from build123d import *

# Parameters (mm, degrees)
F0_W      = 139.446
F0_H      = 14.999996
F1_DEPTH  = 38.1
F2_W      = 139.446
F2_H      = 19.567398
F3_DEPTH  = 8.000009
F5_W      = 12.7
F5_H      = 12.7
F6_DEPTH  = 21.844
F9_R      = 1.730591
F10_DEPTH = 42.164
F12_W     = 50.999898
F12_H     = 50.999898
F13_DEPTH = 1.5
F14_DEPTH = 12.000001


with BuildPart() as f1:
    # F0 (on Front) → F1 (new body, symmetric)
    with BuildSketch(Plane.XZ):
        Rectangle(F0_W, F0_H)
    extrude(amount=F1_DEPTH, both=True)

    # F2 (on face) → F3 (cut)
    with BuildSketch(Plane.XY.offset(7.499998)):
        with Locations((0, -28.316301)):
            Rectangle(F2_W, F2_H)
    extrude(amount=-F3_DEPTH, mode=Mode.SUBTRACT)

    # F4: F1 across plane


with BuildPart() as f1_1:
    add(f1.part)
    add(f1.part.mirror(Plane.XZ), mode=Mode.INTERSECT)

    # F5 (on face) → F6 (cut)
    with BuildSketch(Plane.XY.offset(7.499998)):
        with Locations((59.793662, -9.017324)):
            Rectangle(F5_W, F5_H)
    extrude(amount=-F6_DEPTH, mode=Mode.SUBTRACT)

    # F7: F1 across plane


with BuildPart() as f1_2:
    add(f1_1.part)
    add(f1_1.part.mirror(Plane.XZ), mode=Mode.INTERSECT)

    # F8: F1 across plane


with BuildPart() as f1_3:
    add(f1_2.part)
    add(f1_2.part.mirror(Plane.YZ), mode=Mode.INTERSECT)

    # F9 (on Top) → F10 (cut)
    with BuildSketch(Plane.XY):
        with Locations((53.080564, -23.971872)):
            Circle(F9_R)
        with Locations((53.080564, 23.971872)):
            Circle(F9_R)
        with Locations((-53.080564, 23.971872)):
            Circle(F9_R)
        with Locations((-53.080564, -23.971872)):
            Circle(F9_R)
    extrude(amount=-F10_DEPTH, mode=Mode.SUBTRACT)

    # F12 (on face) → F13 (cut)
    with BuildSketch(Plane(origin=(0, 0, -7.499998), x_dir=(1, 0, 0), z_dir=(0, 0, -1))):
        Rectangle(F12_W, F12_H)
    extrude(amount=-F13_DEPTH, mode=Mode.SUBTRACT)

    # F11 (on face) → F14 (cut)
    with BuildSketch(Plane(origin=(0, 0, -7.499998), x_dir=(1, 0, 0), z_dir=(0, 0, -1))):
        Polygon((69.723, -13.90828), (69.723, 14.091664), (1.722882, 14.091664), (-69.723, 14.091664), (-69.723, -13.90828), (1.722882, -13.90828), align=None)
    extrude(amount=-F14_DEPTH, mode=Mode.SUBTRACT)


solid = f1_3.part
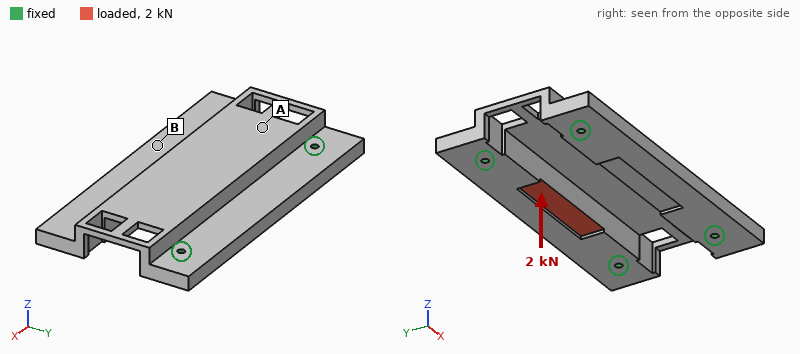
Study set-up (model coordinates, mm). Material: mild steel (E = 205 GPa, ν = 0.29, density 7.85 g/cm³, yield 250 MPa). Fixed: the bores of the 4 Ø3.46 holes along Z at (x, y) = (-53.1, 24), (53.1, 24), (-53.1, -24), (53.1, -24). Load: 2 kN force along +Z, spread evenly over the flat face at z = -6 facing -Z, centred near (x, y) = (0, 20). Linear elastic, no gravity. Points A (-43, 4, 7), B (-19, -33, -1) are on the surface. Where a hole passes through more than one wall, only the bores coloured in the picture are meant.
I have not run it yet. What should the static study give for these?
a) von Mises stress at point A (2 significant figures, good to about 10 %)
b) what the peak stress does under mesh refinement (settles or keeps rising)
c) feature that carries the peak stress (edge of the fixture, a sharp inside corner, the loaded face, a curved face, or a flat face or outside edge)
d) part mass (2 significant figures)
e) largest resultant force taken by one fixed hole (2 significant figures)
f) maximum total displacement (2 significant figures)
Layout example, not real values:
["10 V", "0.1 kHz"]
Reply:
["15 MPa", "keeps rising", "edge of the fixture", "500 g", "1.5 kN", "38 µm"]
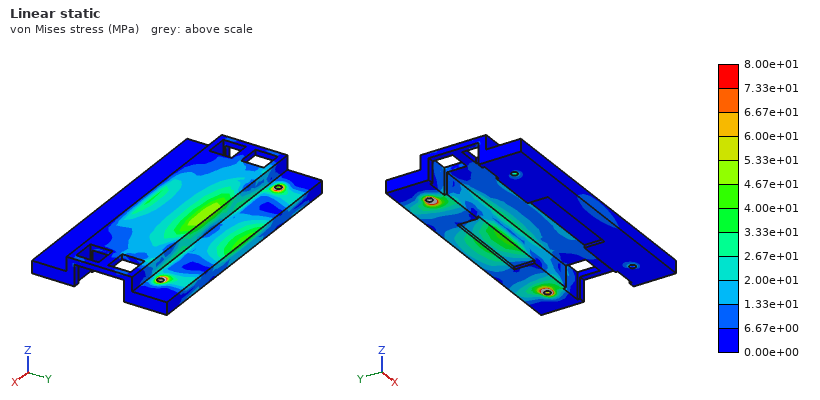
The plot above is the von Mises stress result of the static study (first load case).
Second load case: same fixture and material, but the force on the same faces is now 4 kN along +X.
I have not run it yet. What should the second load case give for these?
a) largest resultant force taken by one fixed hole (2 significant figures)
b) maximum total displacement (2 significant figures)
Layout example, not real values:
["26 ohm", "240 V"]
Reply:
["1.7 kN", "3.8 µm"]
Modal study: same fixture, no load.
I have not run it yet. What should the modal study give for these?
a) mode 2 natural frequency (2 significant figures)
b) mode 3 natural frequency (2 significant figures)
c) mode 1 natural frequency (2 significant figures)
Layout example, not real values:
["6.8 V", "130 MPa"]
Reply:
["3800 Hz", "6500 Hz", "3700 Hz"]
